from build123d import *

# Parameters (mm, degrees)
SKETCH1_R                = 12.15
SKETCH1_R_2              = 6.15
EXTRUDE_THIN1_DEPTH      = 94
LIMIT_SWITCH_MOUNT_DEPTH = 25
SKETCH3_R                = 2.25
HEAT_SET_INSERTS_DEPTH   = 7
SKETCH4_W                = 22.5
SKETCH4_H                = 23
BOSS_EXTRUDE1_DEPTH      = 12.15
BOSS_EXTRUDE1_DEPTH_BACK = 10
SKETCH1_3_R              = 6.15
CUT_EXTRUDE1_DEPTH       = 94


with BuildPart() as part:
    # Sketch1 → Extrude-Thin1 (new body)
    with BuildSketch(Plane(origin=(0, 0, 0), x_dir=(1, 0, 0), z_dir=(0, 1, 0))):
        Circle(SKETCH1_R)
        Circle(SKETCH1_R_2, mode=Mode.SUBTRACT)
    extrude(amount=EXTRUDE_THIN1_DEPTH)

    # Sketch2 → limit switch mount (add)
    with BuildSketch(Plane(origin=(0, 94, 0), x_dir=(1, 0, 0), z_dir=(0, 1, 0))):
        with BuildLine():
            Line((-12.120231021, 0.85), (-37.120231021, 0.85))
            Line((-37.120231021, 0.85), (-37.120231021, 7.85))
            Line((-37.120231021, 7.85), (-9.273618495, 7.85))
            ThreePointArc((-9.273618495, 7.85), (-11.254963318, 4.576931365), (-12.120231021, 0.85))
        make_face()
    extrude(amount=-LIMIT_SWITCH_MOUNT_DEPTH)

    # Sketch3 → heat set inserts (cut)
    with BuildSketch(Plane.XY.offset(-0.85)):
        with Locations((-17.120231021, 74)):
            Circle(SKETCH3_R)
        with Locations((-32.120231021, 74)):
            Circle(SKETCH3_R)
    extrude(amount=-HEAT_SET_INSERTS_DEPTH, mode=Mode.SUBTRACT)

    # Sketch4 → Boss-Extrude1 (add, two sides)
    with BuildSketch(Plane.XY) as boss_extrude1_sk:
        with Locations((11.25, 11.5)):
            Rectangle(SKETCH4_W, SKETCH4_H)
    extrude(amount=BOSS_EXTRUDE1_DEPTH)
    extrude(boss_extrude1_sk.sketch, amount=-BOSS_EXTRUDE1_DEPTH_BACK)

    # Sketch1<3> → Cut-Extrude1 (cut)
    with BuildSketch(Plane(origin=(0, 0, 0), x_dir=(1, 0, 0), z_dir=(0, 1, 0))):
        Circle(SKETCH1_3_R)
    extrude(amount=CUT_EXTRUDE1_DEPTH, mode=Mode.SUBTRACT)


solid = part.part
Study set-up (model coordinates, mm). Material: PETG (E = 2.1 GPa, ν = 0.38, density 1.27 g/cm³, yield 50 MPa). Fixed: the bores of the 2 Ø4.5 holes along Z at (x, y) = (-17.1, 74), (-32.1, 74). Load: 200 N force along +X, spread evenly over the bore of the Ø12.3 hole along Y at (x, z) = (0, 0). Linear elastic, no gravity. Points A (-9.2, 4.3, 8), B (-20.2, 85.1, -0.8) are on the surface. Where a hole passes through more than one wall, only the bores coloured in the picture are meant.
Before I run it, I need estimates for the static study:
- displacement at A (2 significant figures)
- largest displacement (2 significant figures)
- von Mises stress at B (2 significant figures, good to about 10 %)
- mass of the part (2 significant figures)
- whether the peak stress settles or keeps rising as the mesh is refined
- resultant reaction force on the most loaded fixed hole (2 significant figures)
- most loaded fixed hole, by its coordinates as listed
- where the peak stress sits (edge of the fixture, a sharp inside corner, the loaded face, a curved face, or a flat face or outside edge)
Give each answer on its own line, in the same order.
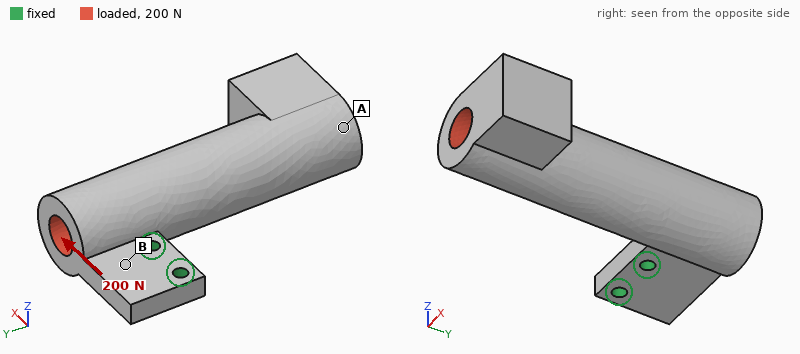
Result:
1.0 mm
1.2 mm
3.3 MPa
55 g
keeps rising
420 N
(-17.1, 74)
edge of the fixture
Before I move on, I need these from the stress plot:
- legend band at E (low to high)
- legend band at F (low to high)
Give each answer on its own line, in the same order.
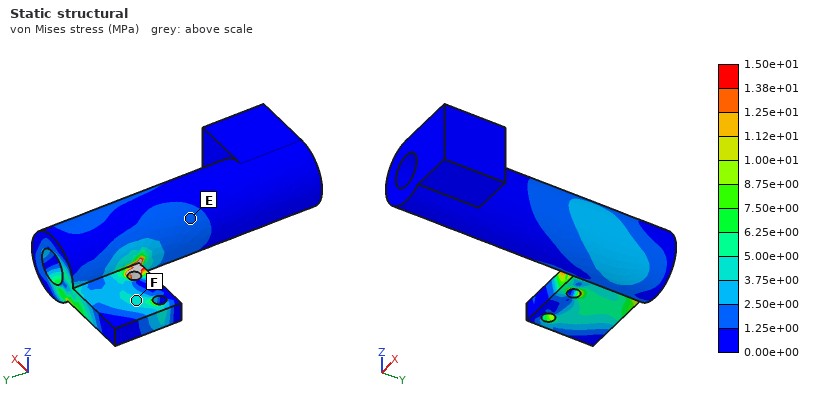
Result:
1.25e+00 to 2.50e+00 MPa
3.75e+00 to 5.00e+00 MPa
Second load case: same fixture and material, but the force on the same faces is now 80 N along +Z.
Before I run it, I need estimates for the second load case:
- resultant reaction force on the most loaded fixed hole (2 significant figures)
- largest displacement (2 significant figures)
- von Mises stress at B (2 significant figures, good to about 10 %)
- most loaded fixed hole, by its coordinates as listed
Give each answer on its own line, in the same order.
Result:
100 N
1.1 mm
3.1 MPa
(-17.1, 74)
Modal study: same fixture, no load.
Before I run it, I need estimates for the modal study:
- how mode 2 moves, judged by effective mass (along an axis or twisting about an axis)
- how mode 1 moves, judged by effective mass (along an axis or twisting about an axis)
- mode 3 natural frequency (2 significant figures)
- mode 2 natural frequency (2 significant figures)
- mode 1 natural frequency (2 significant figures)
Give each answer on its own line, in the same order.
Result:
along X
along Z
630 Hz
310 Hz
210 Hz
